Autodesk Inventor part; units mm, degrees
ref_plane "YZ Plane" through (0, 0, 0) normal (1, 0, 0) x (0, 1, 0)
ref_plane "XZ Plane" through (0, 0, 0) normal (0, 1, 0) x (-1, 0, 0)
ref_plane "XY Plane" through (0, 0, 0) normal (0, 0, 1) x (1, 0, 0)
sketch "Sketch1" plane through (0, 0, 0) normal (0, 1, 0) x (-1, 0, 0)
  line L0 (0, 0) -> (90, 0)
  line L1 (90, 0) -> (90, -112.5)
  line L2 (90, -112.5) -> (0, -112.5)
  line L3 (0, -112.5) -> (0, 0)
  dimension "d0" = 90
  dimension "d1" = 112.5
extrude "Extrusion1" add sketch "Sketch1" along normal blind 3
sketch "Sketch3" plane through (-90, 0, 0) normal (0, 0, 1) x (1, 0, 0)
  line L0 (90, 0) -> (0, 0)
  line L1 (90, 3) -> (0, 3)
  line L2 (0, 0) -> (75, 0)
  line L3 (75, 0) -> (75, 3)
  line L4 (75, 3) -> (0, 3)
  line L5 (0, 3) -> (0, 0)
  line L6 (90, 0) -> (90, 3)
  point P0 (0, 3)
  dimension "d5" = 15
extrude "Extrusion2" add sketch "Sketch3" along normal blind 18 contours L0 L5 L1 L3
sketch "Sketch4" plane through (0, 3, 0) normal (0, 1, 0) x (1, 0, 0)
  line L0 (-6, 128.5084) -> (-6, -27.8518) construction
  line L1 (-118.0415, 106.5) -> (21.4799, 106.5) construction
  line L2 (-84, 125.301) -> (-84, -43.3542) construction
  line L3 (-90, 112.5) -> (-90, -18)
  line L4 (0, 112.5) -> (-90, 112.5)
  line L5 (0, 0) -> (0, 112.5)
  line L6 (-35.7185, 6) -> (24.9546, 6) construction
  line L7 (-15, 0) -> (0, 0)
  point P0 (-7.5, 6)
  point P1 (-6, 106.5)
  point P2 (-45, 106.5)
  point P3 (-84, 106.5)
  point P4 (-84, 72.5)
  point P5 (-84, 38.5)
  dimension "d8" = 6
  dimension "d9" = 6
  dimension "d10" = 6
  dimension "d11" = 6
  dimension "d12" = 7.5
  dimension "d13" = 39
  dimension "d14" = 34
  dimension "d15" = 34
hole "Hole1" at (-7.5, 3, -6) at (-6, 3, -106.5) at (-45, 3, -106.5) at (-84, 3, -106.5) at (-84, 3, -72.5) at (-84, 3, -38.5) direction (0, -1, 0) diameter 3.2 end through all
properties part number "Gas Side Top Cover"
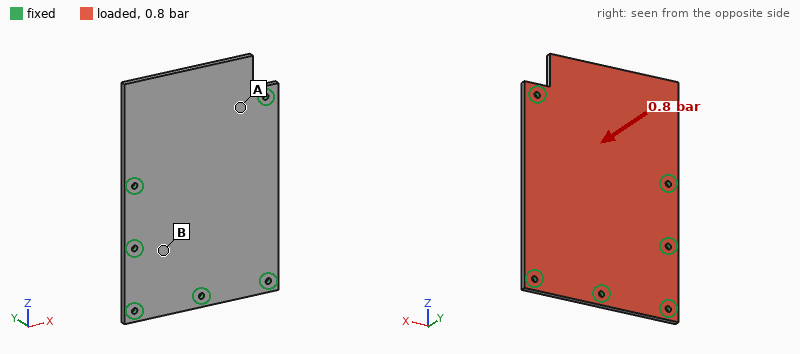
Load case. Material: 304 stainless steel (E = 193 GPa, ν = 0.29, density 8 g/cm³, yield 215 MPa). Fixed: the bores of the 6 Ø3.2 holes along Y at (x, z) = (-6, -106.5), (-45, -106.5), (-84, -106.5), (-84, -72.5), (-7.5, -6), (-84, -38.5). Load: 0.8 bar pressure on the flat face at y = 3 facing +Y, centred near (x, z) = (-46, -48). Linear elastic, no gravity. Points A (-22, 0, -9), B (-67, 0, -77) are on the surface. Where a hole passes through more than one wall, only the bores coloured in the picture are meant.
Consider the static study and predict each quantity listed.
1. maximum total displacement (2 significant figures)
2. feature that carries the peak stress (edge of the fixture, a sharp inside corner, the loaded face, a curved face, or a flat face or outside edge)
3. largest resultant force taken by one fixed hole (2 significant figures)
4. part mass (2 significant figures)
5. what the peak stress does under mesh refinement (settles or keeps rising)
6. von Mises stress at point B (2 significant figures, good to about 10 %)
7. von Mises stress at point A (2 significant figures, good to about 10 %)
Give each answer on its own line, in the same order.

0.17 mm
edge of the fixture
280 N
270 g
keeps rising
11 MPa
37 MPa
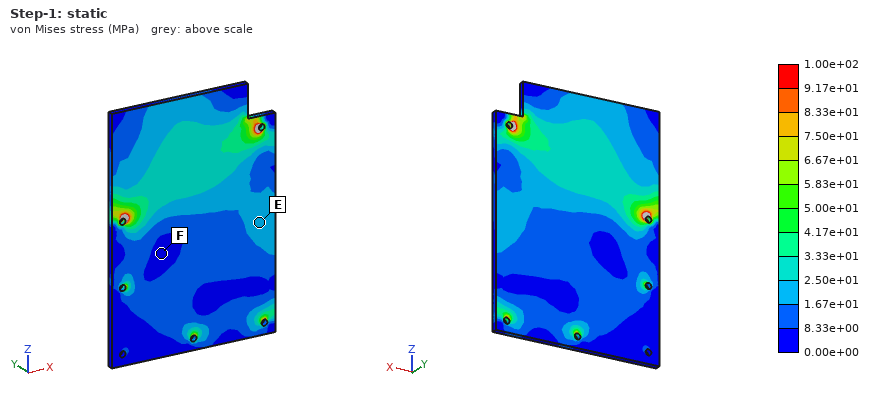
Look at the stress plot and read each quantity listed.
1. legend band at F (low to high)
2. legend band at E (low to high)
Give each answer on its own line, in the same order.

0.00e+00 to 8.33e+00 MPa
1.67e+01 to 2.50e+01 MPa
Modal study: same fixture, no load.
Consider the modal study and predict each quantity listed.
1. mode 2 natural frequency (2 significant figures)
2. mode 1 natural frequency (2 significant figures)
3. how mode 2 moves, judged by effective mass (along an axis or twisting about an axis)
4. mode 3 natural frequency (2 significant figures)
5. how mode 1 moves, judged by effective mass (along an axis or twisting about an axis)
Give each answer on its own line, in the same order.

1500 Hz
890 Hz
along Y
2300 Hz
along Y
